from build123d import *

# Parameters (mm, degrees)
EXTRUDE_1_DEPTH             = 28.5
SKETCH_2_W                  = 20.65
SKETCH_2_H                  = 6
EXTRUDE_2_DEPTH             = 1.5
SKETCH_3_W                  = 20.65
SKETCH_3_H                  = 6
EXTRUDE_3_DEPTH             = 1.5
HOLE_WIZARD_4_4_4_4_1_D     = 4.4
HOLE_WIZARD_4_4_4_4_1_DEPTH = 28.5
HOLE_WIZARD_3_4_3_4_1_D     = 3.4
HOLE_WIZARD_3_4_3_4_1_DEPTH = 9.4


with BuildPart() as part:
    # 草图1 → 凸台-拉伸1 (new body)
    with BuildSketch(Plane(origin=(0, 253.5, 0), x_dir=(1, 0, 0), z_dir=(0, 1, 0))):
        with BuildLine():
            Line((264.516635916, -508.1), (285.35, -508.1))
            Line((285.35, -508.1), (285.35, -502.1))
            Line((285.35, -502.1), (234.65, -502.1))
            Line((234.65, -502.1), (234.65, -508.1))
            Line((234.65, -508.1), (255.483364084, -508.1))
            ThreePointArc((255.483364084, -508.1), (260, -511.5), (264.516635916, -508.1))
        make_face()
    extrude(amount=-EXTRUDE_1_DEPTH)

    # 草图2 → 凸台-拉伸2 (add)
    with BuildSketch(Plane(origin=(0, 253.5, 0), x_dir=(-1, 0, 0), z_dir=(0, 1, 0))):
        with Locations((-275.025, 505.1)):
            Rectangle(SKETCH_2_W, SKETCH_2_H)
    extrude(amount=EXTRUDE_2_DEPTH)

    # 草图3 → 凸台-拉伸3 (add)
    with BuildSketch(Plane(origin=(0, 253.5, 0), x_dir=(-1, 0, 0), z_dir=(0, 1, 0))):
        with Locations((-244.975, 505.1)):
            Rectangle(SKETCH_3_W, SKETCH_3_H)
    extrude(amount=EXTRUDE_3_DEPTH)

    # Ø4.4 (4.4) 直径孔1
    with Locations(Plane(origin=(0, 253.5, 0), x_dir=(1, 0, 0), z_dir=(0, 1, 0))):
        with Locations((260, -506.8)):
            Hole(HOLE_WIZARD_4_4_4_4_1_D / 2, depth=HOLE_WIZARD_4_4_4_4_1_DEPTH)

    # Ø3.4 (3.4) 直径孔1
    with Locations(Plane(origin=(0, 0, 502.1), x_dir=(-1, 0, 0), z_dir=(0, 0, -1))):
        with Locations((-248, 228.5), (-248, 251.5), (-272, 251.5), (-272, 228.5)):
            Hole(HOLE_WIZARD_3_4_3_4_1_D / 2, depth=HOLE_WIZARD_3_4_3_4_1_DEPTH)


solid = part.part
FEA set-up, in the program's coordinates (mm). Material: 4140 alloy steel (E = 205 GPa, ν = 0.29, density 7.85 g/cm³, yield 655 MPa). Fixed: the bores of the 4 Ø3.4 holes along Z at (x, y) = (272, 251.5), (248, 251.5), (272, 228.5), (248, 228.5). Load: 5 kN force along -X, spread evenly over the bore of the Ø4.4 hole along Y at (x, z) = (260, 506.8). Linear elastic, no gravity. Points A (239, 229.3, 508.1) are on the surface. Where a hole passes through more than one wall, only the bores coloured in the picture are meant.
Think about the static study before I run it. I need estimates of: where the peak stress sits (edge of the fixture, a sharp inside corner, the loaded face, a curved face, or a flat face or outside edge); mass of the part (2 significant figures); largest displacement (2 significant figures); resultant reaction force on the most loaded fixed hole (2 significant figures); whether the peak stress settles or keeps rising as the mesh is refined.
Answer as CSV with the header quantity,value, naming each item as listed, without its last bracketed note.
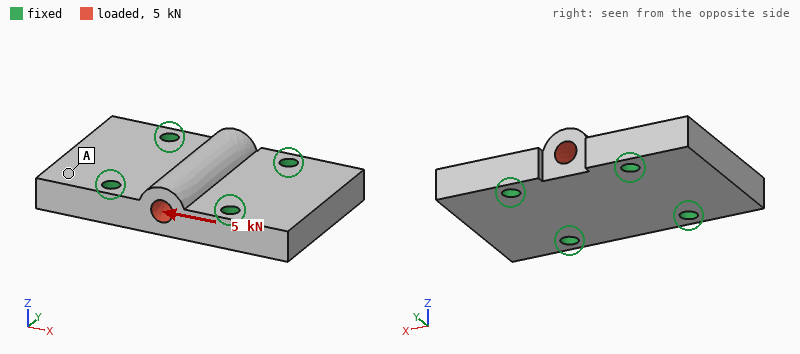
quantity,value
where the peak stress sits,a sharp inside corner
mass of the part,71 g
largest displacement,1.8 µm
resultant reaction force on the most loaded fixed hole,1.3 kN
whether the peak stress settles or keeps rising as the mesh is refined,keeps rising
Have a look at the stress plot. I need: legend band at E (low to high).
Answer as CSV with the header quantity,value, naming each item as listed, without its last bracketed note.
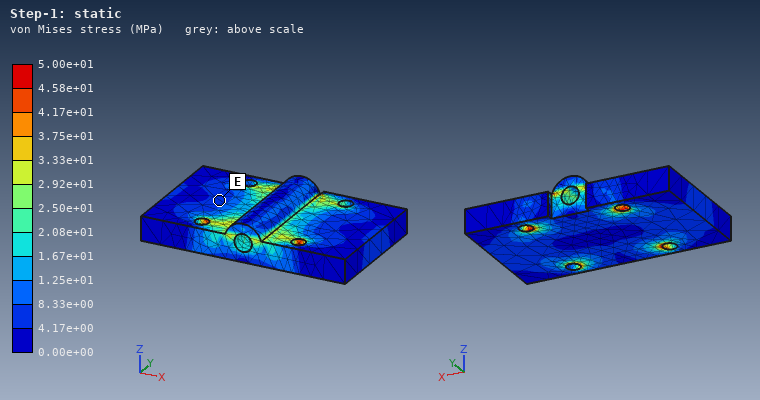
quantity,value
legend band at E,4.17e+00 to 8.33e+00 MPa
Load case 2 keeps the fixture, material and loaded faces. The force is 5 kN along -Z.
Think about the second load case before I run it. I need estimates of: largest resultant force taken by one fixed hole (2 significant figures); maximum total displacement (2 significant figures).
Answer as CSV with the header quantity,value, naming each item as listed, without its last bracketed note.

quantity,value
largest resultant force taken by one fixed hole,1.3 kN
maximum total displacement,6.8 µm
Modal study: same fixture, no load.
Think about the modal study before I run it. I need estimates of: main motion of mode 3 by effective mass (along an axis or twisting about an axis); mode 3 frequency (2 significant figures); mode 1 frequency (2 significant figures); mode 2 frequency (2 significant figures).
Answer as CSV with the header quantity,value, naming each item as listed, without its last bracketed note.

quantity,value
main motion of mode 3 by effective mass,along Z
mode 3 frequency,33 kHz
mode 1 frequency,21 kHz
mode 2 frequency,21 kHz
